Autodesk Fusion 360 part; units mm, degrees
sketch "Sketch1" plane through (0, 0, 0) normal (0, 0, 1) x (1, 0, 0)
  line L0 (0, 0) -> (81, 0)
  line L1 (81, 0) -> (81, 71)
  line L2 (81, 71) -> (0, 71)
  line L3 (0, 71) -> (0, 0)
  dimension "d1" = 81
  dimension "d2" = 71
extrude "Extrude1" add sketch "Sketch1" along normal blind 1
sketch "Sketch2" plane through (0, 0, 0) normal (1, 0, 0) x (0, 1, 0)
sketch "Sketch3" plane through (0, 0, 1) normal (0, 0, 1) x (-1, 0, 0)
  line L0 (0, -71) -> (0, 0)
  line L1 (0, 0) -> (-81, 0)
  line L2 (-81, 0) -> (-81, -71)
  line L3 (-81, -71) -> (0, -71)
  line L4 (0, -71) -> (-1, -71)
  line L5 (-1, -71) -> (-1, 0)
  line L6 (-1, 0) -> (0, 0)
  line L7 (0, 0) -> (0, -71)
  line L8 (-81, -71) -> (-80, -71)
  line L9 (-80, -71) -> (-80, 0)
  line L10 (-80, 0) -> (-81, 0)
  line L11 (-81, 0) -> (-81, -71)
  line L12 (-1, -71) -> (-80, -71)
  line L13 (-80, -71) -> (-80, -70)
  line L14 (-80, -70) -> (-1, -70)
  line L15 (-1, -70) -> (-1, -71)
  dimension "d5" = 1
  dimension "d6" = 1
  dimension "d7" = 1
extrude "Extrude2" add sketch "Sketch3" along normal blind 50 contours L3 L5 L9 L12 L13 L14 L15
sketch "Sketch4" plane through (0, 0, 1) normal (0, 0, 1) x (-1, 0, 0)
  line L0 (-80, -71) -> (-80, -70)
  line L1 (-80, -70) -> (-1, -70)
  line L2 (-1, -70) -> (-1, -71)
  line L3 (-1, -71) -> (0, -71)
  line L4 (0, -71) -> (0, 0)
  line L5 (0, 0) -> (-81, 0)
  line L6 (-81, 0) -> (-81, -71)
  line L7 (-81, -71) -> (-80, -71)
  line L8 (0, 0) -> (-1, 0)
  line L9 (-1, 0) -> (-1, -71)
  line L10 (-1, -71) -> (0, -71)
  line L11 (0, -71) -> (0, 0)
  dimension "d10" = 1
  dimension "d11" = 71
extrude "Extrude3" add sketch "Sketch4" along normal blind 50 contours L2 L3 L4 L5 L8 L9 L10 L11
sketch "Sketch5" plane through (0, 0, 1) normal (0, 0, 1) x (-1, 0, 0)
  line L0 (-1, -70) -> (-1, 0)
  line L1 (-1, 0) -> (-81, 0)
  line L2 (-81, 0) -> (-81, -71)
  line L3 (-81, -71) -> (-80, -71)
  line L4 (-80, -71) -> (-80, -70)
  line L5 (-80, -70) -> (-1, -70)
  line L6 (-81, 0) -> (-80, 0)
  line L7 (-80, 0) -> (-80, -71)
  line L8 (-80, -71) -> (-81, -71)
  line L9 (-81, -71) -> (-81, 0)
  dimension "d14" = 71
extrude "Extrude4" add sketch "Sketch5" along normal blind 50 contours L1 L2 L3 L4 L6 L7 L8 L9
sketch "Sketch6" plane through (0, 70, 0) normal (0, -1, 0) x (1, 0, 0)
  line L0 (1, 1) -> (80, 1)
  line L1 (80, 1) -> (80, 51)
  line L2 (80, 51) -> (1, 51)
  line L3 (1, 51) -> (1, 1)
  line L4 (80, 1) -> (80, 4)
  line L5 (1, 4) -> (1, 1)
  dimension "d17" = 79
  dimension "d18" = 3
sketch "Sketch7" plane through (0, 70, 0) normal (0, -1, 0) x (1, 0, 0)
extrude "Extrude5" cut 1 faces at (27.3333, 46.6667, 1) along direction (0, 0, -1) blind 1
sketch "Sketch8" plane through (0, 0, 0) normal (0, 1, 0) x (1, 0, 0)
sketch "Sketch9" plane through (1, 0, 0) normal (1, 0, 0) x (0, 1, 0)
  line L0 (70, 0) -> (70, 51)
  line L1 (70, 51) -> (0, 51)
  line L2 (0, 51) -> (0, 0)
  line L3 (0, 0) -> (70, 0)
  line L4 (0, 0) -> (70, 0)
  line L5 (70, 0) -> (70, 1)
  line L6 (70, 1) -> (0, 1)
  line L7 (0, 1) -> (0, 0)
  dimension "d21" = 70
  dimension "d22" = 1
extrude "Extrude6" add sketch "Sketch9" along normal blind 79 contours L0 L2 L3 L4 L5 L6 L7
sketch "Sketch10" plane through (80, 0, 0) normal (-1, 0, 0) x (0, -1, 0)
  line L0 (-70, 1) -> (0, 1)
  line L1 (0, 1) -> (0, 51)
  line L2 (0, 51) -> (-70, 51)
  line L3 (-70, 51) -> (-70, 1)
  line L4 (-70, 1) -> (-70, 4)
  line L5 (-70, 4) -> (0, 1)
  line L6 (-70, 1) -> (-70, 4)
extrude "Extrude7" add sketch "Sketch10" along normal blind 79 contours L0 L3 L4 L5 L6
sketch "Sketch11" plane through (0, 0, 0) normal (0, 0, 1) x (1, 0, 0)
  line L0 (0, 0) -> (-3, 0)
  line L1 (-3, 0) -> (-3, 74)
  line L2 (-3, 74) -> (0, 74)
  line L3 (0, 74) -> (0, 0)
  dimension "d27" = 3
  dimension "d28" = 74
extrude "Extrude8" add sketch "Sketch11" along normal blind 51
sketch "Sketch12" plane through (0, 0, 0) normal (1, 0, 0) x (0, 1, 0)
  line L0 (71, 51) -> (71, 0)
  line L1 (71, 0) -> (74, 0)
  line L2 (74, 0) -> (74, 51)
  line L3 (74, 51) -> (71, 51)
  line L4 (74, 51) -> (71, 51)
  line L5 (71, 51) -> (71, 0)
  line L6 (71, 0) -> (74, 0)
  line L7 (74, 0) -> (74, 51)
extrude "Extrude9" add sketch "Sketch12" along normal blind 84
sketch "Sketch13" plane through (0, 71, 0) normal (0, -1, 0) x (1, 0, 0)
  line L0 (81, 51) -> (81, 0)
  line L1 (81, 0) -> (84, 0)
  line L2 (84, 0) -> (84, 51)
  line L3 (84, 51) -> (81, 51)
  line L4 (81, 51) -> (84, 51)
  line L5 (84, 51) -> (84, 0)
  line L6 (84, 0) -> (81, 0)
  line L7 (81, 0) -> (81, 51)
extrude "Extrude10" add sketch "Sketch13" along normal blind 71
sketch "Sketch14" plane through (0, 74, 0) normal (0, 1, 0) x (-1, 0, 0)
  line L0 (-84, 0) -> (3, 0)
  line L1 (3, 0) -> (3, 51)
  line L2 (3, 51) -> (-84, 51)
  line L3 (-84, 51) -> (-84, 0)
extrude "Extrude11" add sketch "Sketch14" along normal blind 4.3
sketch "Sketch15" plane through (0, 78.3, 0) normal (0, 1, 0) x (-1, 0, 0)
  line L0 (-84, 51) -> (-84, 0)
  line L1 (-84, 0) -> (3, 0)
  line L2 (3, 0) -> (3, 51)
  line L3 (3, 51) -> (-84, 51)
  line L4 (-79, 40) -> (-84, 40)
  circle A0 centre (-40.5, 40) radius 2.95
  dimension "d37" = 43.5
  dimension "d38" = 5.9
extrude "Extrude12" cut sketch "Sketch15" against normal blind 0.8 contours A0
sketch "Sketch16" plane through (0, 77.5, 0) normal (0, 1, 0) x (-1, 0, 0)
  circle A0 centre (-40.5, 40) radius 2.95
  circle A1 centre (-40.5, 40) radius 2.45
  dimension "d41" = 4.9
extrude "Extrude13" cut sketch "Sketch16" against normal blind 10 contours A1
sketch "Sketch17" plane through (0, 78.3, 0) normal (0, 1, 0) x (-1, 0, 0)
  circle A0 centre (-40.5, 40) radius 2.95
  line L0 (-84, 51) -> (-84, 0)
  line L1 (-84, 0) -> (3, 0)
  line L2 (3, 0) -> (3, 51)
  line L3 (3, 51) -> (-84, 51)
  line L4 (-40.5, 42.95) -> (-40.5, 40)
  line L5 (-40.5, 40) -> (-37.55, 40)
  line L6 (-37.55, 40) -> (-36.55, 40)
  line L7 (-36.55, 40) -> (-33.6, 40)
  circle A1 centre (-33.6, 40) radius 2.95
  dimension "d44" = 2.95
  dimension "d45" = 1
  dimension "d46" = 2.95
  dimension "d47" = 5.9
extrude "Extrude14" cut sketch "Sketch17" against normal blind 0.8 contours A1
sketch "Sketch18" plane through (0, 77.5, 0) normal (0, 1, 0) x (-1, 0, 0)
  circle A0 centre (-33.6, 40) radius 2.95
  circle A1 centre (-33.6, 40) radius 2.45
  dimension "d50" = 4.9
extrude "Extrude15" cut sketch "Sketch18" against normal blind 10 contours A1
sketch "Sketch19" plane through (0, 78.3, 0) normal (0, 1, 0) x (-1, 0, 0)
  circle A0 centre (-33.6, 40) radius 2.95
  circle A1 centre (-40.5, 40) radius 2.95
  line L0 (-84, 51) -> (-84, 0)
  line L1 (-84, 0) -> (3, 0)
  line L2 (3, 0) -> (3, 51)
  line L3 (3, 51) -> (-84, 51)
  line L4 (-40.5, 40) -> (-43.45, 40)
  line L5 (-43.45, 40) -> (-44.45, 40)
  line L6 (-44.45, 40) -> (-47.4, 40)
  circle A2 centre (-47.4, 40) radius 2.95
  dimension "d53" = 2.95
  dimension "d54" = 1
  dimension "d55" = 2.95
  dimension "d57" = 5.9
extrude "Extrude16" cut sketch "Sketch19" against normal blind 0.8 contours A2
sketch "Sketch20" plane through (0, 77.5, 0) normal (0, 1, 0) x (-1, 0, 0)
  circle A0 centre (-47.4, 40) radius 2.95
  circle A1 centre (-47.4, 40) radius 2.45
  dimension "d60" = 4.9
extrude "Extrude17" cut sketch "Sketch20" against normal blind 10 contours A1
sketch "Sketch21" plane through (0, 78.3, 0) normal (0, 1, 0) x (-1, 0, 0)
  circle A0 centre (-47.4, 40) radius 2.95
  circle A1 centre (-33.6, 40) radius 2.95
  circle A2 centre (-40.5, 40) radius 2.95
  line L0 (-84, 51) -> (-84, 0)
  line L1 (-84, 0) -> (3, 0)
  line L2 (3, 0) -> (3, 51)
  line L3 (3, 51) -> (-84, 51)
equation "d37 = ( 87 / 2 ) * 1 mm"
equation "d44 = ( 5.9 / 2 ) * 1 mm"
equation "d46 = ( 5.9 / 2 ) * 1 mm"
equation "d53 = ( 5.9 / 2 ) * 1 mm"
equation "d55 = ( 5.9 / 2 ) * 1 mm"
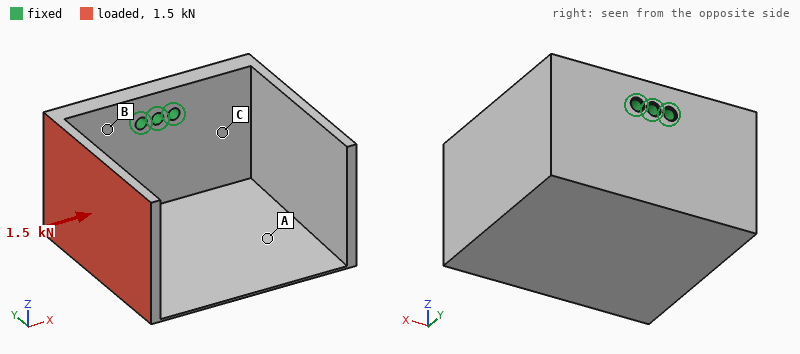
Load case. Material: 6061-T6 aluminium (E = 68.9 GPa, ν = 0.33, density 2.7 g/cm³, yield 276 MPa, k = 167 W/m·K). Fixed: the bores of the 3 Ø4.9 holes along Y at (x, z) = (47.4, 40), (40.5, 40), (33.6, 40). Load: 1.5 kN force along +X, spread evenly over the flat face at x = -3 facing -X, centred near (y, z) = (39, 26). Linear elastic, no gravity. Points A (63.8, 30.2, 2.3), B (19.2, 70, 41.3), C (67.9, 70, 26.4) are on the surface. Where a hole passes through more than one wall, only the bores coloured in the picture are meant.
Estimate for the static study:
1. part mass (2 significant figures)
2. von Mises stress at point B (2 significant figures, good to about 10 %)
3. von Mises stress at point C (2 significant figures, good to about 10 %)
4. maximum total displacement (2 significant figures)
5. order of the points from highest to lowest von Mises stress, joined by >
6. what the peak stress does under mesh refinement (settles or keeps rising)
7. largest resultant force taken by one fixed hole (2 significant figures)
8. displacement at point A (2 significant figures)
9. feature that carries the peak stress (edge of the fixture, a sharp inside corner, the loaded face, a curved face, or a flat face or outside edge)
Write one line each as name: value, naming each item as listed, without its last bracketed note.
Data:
part mass: 210 g
von Mises stress at point B: 55 MPa
von Mises stress at point C: 24 MPa
maximum total displacement: 1.5 mm
order of the points from highest to lowest von Mises stress, joined by >: B > C > A
what the peak stress does under mesh refinement: keeps rising
largest resultant force taken by one fixed hole: 2.3 kN
displacement at point A: 0.29 mm
feature that carries the peak stress: edge of the fixture
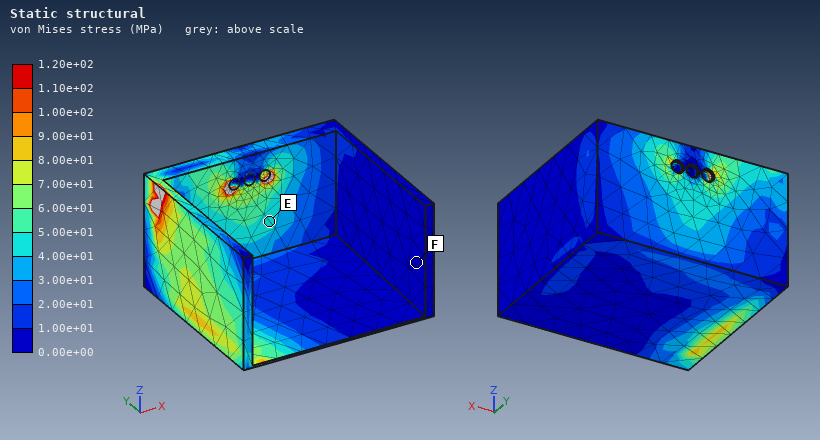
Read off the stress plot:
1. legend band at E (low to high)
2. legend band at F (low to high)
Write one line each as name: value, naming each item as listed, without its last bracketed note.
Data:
legend band at E: 4.00e+01 to 5.00e+01 MPa
legend band at F: 0.00e+00 to 1.00e+01 MPa
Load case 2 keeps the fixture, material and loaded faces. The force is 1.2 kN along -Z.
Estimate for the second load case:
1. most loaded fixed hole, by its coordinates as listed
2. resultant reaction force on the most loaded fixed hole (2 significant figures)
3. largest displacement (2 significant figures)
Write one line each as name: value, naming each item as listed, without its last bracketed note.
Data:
most loaded fixed hole, by its coordinates as listed: (33.6, 40)
resultant reaction force on the most loaded fixed hole: 3.3 kN
largest displacement: 0.62 mm
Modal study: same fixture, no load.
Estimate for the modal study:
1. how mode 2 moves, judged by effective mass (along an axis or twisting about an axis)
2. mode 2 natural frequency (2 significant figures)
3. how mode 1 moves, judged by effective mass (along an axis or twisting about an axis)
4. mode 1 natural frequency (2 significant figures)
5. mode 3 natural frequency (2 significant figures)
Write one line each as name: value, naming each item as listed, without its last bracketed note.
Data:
how mode 2 moves, judged by effective mass: along Z
mode 2 natural frequency: 920 Hz
how mode 1 moves, judged by effective mass: along X
mode 1 natural frequency: 780 Hz
mode 3 natural frequency: 1200 Hz
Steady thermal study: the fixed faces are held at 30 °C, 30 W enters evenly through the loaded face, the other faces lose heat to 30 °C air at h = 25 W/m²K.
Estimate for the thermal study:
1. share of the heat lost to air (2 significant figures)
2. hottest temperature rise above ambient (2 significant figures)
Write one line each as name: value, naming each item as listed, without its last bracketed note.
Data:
share of the heat lost to air: 24 %
hottest temperature rise above ambient: 29 K
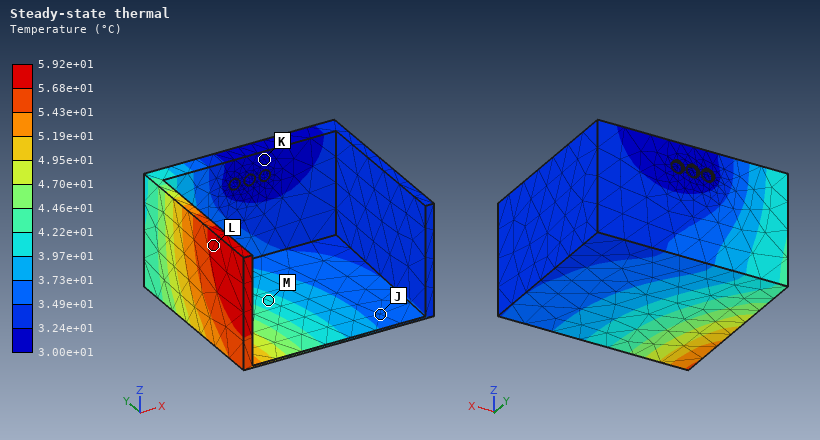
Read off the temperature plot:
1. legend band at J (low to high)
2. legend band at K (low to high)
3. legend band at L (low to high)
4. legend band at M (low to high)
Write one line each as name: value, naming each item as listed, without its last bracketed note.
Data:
legend band at J: 3.49e+01 to 3.73e+01 °C
legend band at K: 3.00e+01 to 3.24e+01 °C
legend band at L: 5.68e+01 to 5.92e+01 °C
legend band at M: 3.97e+01 to 4.22e+01 °C
